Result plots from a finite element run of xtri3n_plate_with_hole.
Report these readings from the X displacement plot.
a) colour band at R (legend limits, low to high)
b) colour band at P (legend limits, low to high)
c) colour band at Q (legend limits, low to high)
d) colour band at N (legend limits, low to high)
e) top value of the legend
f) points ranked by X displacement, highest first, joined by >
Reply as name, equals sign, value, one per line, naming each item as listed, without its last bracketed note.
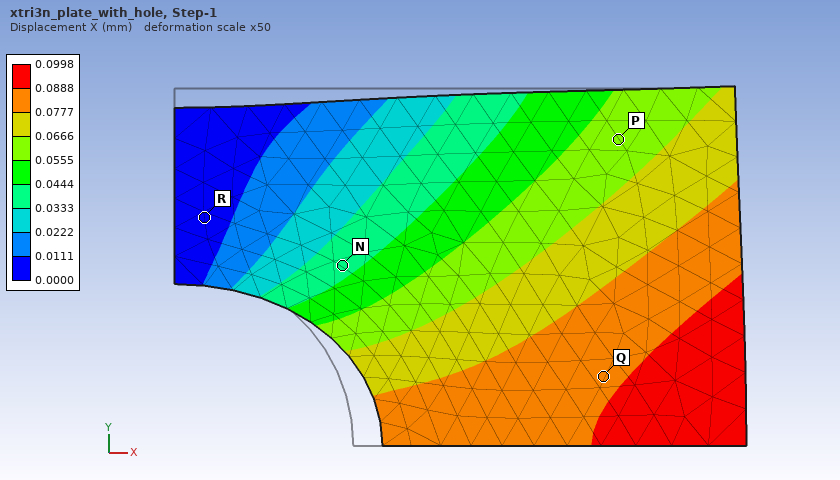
colour band at R = 0.0000 to 0.0111 mm
colour band at P = 0.0555 to 0.0666 mm
colour band at Q = 0.0777 to 0.0888 mm
colour band at N = 0.0333 to 0.0444 mm
top value of the legend = 0.0998 mm
points ranked by X displacement, highest first, joined by > = Q > P > N > R
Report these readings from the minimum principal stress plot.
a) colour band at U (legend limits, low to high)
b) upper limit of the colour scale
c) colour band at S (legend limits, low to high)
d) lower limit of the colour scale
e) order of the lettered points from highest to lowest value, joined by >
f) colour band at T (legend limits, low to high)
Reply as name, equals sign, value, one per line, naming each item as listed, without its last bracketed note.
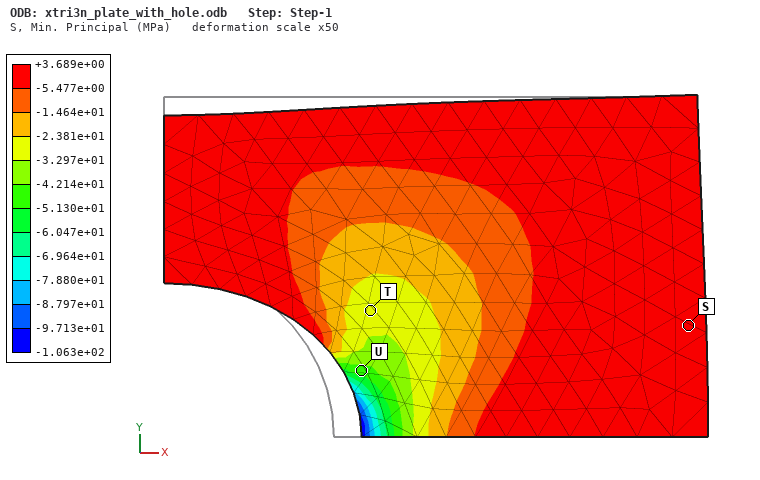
colour band at U = -5.130e+01 to -4.214e+01 MPa
upper limit of the colour scale = +3.689e+00 MPa
colour band at S = -5.477e+00 to +3.689e+00 MPa
lower limit of the colour scale = -1.063e+02 MPa
order of the lettered points from highest to lowest value, joined by > = S > T > U
colour band at T = -3.297e+01 to -2.381e+01 MPa
